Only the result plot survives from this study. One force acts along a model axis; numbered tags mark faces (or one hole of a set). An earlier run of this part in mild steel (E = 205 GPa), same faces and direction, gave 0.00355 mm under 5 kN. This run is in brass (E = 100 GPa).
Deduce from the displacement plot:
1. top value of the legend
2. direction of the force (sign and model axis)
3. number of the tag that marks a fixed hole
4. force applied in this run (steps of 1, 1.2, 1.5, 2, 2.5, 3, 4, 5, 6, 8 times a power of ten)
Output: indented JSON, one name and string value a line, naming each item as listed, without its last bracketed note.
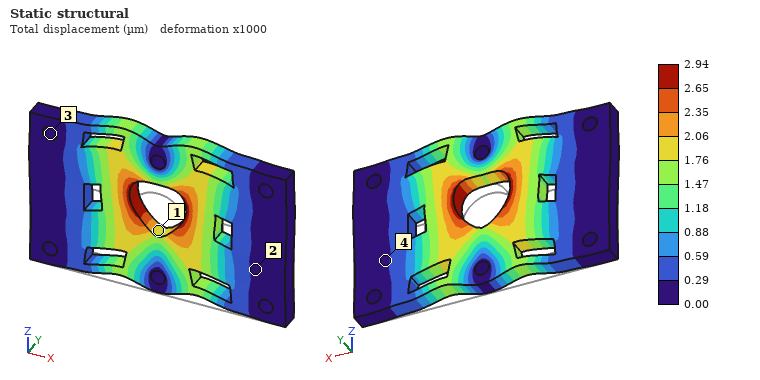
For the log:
{
  "top value of the legend": "2.94 µm",
  "direction of the force": "+Z",
  "number of the tag that marks a fixed hole": "3",
  "force applied in this run": "2 kN"
}
